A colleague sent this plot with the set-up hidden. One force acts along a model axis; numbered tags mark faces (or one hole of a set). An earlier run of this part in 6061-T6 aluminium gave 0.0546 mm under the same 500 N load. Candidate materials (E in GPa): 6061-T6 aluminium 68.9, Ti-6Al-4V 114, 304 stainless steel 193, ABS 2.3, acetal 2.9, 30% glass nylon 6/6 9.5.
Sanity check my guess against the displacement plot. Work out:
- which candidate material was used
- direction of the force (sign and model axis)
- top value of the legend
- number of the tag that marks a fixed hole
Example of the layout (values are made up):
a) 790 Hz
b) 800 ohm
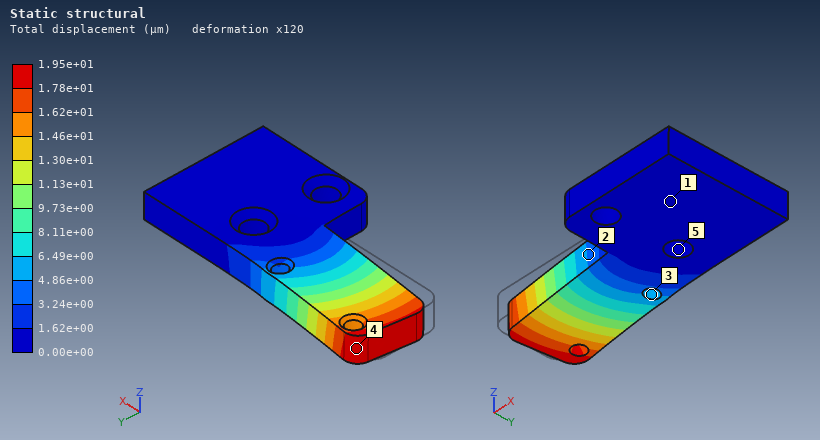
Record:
a) 304 stainless steel
b) +Y
c) 1.95e+01 µm
d) 5
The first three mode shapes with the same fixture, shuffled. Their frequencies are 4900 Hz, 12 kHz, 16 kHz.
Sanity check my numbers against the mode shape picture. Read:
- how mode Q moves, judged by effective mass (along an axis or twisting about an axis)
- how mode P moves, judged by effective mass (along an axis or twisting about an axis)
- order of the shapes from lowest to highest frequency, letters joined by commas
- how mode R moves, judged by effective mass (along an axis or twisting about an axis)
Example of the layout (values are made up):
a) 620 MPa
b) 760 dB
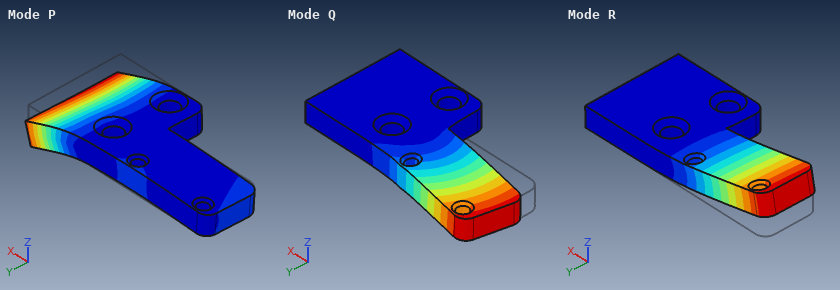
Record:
a) along Y
b) along Z
c) R, Q, P
d) along Z
